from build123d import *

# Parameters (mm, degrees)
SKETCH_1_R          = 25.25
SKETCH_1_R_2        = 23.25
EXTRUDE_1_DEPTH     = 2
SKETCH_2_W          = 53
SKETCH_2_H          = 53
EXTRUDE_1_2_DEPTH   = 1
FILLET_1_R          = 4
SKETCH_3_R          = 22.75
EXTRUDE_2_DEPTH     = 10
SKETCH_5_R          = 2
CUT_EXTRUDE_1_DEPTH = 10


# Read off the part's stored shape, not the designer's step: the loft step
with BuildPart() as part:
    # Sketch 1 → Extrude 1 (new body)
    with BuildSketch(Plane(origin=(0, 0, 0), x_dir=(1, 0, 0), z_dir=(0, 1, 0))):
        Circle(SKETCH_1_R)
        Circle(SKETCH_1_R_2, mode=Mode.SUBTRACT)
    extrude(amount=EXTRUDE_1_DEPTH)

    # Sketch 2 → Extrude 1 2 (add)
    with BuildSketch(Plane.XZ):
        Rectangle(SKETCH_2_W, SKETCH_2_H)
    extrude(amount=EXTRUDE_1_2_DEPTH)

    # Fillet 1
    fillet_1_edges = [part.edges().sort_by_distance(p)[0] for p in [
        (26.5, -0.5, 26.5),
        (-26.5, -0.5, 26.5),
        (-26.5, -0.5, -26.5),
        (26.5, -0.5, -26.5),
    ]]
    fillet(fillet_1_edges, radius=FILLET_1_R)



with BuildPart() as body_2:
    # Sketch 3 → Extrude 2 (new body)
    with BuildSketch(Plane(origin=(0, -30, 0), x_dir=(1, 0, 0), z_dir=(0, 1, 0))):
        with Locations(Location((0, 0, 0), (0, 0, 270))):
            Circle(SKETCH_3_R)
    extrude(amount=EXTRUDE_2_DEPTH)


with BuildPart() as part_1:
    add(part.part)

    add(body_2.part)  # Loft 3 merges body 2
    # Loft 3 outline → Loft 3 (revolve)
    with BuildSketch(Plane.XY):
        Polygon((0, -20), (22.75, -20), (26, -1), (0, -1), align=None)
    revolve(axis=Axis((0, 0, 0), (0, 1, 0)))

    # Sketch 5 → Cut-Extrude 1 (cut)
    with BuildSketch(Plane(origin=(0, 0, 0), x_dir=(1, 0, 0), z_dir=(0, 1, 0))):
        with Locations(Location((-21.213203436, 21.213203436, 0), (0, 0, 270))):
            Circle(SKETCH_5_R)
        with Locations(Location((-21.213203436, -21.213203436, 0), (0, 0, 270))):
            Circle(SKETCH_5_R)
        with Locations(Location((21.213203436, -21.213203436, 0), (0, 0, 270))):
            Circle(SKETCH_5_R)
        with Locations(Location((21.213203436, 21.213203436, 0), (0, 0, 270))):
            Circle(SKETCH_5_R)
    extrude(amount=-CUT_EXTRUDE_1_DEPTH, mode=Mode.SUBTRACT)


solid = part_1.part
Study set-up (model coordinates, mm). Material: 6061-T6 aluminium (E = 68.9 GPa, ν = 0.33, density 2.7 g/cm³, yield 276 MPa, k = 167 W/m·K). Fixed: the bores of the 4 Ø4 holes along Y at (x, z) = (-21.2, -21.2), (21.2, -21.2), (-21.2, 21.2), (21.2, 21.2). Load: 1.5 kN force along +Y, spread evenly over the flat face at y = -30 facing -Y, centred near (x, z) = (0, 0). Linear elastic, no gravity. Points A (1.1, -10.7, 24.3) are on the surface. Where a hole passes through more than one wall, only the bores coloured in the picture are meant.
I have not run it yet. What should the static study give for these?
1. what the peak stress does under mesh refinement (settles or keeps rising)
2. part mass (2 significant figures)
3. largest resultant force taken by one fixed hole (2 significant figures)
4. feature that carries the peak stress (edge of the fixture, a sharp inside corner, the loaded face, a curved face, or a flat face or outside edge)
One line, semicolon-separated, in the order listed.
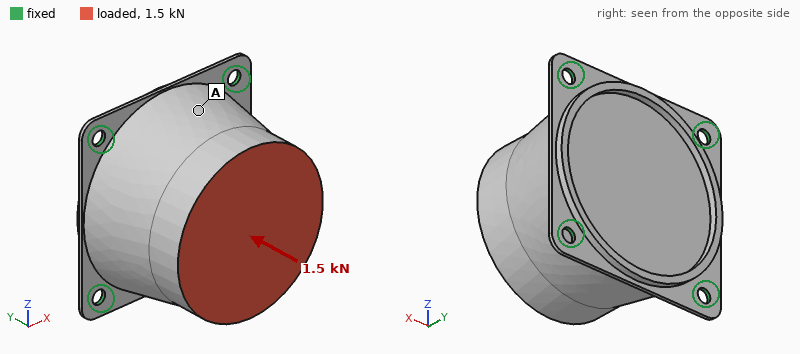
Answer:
keeps rising; 150 g; 440 N; edge of the fixture
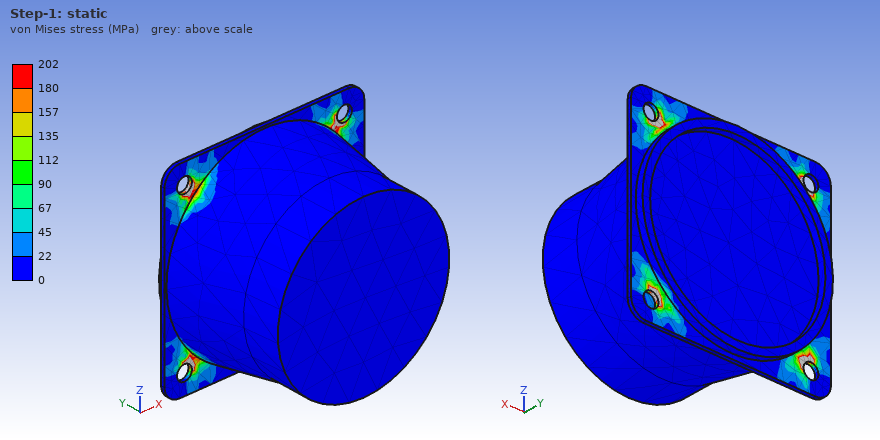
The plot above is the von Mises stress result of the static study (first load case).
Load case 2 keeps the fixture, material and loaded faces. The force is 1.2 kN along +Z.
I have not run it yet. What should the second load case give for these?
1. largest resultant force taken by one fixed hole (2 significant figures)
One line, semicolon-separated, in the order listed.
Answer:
590 N
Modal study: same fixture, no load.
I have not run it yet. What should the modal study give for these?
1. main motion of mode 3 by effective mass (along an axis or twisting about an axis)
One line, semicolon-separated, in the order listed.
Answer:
along Y
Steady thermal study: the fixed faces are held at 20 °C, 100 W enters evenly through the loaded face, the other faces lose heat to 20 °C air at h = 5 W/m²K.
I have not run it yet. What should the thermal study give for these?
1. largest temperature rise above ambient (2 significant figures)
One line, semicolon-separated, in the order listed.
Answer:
64 K
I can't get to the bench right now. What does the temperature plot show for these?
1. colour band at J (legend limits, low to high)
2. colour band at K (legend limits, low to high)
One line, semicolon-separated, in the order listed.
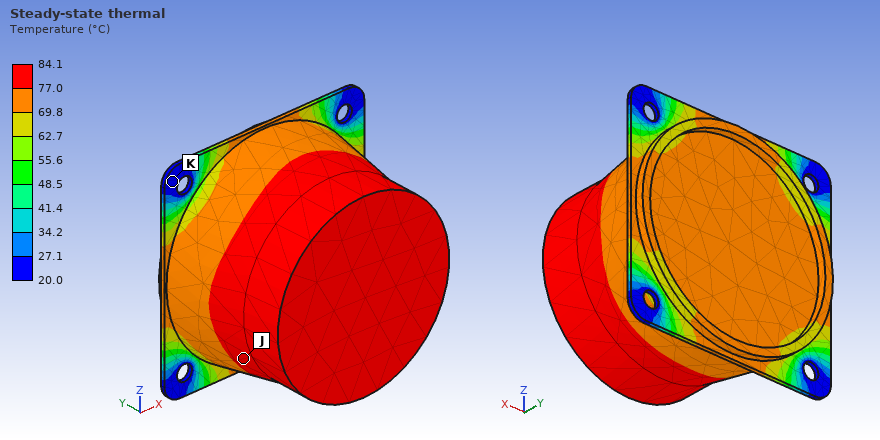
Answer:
77.0 to 84.1 °C; 20.0 to 27.1 °C
